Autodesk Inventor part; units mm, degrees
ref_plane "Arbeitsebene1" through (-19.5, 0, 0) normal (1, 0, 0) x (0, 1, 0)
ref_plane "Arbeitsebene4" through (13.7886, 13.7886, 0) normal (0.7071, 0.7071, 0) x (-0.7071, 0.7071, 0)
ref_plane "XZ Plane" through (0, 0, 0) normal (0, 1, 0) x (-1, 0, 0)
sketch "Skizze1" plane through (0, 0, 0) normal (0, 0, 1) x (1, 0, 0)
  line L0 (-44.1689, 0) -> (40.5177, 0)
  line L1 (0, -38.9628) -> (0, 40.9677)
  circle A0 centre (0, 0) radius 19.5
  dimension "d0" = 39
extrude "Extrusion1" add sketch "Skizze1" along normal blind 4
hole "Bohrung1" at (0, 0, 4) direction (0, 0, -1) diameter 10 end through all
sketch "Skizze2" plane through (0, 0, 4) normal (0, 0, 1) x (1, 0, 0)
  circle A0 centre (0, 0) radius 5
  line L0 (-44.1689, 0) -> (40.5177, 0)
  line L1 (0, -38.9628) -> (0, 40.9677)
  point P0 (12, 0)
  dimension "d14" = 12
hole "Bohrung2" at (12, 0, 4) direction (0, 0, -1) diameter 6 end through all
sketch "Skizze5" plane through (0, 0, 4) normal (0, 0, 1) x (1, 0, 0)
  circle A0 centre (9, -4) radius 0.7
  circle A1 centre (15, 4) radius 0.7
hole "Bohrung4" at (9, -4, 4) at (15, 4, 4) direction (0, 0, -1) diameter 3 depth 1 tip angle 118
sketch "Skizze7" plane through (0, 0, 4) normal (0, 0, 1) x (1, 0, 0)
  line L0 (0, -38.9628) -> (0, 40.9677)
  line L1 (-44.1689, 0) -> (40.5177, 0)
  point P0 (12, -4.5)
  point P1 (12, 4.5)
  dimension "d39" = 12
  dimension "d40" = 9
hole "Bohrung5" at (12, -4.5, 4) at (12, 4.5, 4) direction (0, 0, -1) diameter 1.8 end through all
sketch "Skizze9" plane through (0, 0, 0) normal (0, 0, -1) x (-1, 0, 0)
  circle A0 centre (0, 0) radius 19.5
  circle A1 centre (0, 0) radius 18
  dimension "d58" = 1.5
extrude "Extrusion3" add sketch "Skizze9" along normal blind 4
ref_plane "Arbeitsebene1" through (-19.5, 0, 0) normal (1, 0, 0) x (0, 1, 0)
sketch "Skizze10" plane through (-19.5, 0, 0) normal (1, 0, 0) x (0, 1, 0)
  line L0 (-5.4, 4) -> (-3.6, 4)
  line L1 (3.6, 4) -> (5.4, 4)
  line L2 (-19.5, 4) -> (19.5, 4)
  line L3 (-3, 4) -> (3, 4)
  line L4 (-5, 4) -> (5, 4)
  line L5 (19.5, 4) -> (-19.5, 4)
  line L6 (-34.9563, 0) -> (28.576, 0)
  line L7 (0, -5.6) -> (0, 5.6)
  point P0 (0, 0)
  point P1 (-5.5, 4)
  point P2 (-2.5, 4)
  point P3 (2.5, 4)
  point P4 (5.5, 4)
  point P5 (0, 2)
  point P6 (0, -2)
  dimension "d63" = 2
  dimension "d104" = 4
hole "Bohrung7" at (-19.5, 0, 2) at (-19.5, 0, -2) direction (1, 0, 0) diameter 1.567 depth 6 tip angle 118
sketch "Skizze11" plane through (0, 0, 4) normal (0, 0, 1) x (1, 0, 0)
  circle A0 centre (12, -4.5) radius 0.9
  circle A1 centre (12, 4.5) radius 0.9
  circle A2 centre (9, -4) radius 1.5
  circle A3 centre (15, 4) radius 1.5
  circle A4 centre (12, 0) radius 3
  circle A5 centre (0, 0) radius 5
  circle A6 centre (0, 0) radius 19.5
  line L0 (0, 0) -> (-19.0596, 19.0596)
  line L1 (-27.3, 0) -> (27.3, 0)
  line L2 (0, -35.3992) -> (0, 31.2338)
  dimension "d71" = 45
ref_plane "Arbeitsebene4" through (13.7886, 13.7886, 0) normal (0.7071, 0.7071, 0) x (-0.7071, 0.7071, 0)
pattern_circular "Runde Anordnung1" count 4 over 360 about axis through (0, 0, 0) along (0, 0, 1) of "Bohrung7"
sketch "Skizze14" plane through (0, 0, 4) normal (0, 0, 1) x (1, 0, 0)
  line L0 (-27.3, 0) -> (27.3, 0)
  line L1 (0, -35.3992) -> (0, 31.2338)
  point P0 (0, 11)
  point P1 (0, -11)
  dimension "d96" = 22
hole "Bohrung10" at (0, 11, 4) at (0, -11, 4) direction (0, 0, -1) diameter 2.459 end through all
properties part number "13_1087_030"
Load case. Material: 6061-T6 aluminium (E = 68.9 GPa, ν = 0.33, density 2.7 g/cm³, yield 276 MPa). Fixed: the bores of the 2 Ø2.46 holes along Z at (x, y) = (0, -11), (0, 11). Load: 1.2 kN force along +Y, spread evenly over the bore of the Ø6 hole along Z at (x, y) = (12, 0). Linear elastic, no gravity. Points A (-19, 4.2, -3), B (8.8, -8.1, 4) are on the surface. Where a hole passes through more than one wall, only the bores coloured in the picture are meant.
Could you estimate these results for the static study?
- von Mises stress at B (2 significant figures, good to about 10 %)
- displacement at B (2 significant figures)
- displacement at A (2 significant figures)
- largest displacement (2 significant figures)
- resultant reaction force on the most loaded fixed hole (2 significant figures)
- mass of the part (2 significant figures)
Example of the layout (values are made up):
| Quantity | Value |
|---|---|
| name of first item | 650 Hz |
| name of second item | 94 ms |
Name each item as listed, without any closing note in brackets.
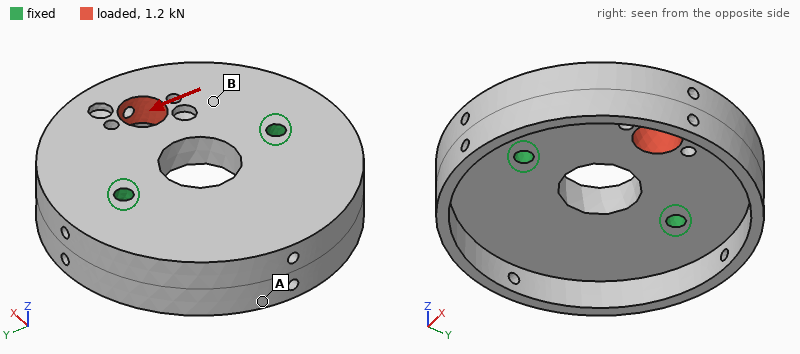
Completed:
| Quantity | Value |
|---|---|
| von Mises stress at B | 14 MPa |
| displacement at B | 6.7 µm |
| displacement at A | 2.5 µm |
| largest displacement | 13 µm |
| resultant reaction force on the most loaded fixed hole | 830 N |
| mass of the part | 13 g |
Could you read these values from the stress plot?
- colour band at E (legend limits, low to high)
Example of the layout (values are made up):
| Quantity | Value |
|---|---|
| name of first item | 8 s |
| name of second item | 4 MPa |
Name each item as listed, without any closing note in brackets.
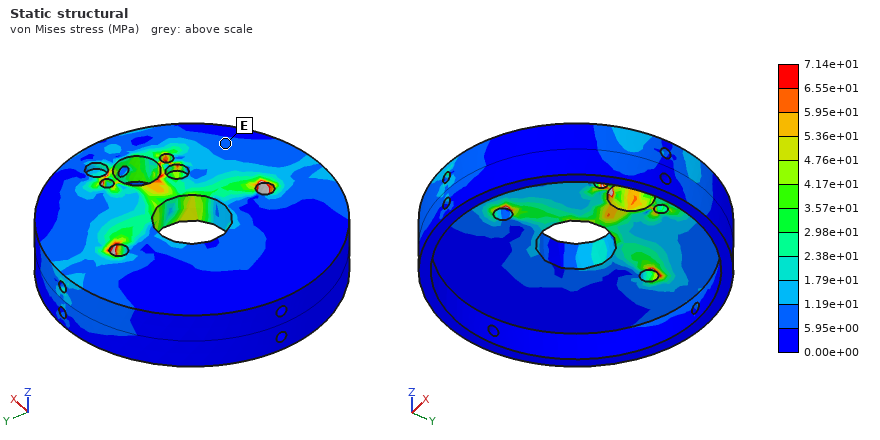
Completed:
| Quantity | Value |
|---|---|
| colour band at E | 5.95e+00 to 1.19e+01 MPa |
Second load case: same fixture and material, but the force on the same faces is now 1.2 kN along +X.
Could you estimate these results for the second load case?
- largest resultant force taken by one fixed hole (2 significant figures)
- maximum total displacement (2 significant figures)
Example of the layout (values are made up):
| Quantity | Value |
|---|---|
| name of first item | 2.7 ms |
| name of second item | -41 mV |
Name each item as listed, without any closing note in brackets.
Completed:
| Quantity | Value |
|---|---|
| largest resultant force taken by one fixed hole | 650 N |
| maximum total displacement | 7.3 µm |
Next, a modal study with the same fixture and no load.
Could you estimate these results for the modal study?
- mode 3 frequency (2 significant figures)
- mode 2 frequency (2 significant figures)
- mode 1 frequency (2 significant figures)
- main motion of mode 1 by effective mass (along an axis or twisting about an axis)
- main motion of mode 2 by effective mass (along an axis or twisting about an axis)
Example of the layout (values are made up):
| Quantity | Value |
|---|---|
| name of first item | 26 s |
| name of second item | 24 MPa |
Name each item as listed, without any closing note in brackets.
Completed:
| Quantity | Value |
|---|---|
| mode 3 frequency | 16 kHz |
| mode 2 frequency | 10 kHz |
| mode 1 frequency | 7500 Hz |
| main motion of mode 1 by effective mass | twisting about Y |
| main motion of mode 2 by effective mass | along Z |
